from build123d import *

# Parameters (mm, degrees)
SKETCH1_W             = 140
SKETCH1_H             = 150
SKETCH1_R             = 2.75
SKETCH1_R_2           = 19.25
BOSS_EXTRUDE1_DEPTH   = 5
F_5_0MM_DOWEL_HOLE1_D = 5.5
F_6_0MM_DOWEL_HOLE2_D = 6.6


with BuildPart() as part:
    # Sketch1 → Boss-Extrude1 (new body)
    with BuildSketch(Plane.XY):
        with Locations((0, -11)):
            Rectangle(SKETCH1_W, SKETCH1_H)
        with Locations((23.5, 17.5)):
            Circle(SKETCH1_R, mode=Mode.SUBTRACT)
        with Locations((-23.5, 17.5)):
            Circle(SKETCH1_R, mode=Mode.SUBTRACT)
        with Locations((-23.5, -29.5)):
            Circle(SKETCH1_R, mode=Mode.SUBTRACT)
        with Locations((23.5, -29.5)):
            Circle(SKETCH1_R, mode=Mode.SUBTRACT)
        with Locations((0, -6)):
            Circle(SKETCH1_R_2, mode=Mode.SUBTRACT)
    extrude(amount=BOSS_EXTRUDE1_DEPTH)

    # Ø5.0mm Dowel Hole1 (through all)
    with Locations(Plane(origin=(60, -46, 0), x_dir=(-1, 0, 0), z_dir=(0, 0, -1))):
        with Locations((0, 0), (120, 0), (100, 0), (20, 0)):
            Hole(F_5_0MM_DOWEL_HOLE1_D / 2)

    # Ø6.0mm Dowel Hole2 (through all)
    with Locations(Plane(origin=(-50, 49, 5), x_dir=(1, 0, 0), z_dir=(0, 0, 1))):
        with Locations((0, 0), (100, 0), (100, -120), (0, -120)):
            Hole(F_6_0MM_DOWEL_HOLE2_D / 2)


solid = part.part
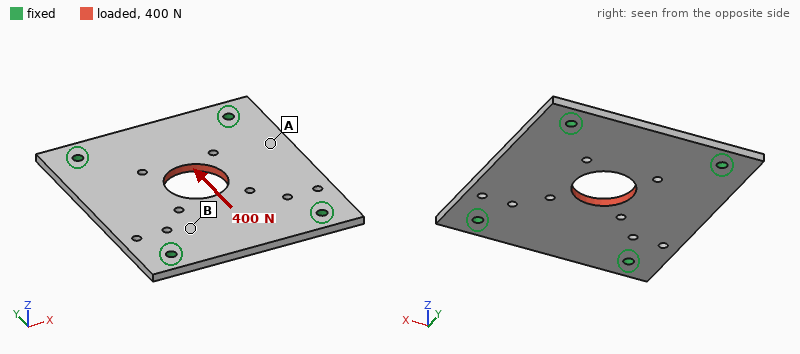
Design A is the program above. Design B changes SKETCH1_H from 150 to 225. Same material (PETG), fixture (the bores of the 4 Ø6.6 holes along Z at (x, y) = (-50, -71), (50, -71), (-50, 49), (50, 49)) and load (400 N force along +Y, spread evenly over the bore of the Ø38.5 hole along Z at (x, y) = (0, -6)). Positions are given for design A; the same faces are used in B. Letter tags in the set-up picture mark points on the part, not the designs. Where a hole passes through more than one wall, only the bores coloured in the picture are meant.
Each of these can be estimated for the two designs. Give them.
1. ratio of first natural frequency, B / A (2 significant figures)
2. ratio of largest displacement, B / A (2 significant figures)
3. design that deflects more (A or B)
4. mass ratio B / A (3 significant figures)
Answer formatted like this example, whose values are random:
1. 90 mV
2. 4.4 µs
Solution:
1. 0.78
2. 0.79
3. A
4. 1.54
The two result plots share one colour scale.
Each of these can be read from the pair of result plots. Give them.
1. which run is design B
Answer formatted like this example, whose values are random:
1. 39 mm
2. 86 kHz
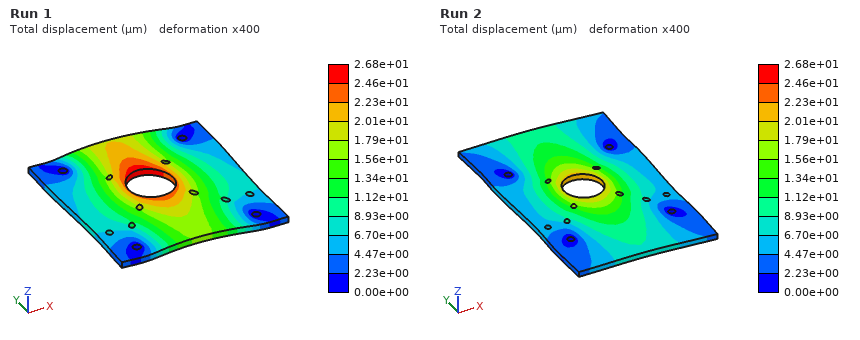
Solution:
1. Run 2
